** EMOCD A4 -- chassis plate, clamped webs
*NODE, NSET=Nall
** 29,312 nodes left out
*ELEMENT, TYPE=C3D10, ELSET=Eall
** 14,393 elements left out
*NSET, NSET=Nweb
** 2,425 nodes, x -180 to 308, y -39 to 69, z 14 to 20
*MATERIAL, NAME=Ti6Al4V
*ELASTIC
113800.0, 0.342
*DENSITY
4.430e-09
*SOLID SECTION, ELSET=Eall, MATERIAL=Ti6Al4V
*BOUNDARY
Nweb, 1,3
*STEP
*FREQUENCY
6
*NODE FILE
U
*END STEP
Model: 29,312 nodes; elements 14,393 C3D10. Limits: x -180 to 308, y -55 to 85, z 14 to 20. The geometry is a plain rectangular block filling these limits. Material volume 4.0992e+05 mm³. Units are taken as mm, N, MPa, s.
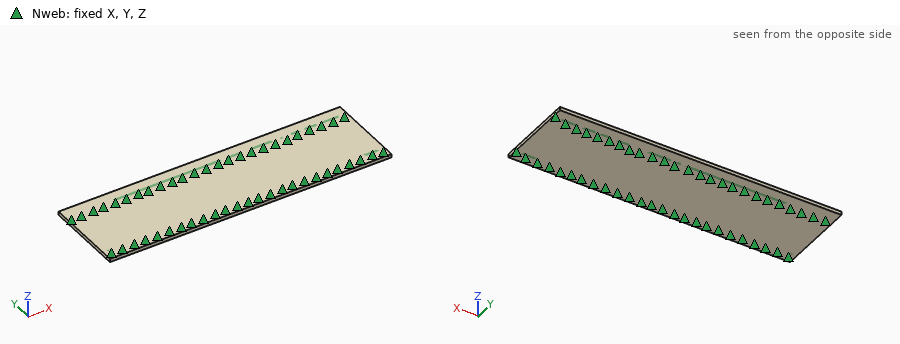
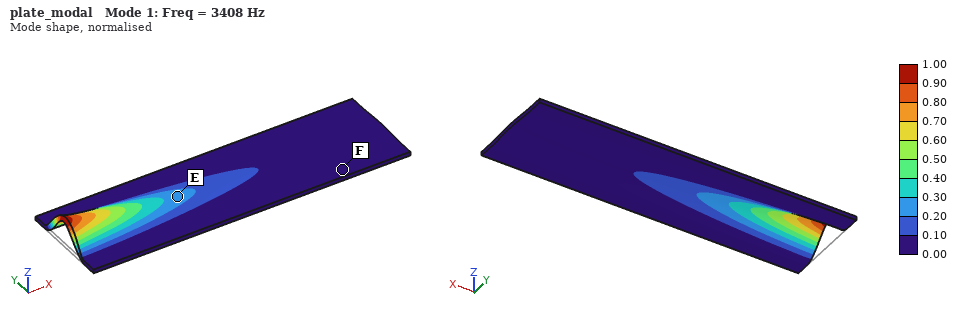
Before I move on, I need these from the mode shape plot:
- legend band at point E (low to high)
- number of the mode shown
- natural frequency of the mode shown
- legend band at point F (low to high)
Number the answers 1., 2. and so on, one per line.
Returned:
1. 0.20 to 0.30
2. 1
3. 3408 Hz
4. 0.00 to 0.10
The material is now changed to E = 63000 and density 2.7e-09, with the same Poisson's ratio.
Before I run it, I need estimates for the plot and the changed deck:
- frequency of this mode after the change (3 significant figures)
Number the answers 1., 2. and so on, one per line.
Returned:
1. 3250 Hz
